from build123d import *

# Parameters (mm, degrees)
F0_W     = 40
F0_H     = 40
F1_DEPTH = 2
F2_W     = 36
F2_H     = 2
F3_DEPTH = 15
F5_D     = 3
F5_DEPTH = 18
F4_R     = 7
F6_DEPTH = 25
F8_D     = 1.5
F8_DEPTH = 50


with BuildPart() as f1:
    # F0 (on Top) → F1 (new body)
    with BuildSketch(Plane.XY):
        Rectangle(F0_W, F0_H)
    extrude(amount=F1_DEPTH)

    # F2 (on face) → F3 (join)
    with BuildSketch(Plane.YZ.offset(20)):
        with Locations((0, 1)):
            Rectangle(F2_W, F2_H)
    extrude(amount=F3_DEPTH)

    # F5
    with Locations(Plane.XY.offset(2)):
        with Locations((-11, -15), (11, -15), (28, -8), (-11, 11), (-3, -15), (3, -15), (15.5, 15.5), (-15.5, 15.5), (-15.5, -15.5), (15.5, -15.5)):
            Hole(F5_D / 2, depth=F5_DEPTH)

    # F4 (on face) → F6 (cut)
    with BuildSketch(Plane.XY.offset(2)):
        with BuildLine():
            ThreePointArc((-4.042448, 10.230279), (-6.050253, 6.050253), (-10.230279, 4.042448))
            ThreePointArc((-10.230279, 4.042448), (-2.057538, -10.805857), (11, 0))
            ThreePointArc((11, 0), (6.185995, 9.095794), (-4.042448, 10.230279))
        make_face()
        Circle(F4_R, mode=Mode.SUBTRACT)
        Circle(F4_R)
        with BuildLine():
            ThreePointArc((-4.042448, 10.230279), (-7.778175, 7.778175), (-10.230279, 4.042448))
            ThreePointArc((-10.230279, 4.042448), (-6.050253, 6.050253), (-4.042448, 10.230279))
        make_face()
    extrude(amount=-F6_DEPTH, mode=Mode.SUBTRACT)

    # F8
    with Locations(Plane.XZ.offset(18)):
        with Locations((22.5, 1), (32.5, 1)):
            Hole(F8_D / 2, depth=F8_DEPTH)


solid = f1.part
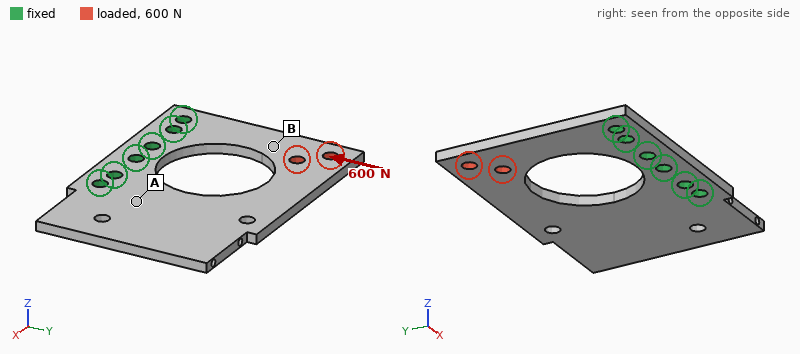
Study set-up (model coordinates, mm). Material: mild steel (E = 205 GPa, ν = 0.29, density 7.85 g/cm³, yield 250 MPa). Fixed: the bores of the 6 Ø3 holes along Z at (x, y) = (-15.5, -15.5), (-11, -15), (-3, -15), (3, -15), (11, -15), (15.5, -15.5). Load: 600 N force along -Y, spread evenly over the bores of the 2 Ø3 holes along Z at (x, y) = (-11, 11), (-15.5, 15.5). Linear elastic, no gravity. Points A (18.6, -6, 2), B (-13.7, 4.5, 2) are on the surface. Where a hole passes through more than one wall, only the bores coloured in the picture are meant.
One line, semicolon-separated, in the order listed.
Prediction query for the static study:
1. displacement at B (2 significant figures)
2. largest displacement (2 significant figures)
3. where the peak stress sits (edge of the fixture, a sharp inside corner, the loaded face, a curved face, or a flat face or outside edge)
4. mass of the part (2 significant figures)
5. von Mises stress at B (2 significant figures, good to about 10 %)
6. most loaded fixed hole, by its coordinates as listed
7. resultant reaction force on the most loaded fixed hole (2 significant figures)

3.1 µm; 4.8 µm; the loaded face; 26 g; 30 MPa; (-15.5, -15.5); 410 N
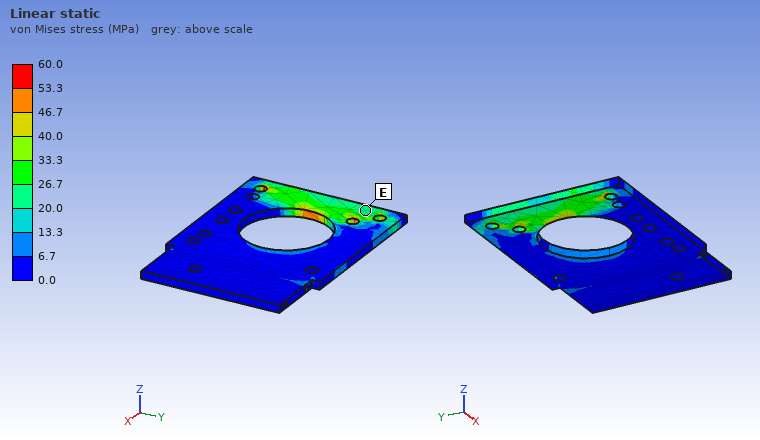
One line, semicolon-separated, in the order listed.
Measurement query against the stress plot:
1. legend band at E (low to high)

20.0 to 26.7 MPa
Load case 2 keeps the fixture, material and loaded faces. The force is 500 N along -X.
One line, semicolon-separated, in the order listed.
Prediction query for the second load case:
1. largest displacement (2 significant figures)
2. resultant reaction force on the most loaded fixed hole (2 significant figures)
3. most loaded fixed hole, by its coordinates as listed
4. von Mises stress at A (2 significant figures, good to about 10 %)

16 µm; 570 N; (15.5, -15.5); 24 MPa
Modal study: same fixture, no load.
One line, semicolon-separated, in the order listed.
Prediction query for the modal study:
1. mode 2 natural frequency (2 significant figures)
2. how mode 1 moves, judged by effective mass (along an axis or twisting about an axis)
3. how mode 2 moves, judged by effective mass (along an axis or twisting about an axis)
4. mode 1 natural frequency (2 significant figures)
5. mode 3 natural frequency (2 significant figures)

1900 Hz; along Z; twisting about Y; 1100 Hz; 4100 Hz
